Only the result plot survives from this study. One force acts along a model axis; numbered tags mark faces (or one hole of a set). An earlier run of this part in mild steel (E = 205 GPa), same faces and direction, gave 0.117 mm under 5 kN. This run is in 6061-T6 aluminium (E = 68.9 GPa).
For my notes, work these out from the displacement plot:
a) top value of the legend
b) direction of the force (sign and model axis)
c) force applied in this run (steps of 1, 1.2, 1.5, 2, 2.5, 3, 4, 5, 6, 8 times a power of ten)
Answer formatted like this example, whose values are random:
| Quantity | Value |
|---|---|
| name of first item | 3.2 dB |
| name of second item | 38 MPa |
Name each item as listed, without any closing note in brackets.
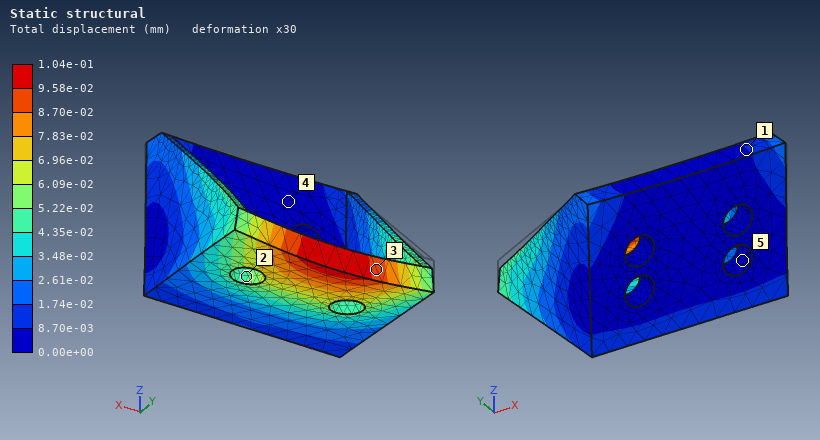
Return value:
| Quantity | Value |
|---|---|
| top value of the legend | 1.04e-01 mm |
| direction of the force | -Z |
| force applied in this run | 1.5 kN |
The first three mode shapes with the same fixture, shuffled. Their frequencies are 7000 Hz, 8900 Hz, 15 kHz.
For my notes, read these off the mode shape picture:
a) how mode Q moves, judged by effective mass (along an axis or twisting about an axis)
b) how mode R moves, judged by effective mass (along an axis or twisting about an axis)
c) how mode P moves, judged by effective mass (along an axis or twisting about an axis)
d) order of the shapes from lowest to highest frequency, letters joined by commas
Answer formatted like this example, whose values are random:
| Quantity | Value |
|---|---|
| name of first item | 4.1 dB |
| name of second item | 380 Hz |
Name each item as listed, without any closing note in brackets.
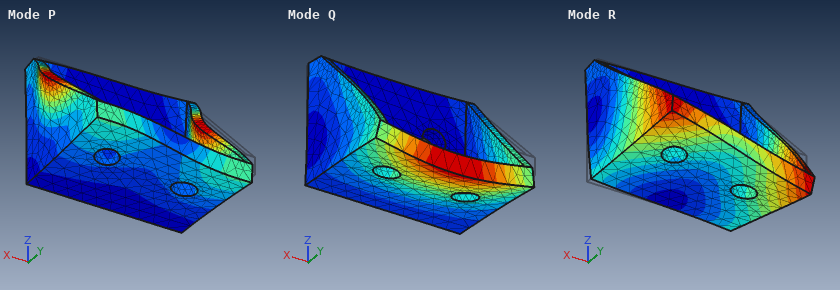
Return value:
| Quantity | Value |
|---|---|
| how mode Q moves, judged by effective mass | along Z |
| how mode R moves, judged by effective mass | along X |
| how mode P moves, judged by effective mass | along X |
| order of the shapes from lowest to highest frequency, letters joined by commas | Q, R, P |
